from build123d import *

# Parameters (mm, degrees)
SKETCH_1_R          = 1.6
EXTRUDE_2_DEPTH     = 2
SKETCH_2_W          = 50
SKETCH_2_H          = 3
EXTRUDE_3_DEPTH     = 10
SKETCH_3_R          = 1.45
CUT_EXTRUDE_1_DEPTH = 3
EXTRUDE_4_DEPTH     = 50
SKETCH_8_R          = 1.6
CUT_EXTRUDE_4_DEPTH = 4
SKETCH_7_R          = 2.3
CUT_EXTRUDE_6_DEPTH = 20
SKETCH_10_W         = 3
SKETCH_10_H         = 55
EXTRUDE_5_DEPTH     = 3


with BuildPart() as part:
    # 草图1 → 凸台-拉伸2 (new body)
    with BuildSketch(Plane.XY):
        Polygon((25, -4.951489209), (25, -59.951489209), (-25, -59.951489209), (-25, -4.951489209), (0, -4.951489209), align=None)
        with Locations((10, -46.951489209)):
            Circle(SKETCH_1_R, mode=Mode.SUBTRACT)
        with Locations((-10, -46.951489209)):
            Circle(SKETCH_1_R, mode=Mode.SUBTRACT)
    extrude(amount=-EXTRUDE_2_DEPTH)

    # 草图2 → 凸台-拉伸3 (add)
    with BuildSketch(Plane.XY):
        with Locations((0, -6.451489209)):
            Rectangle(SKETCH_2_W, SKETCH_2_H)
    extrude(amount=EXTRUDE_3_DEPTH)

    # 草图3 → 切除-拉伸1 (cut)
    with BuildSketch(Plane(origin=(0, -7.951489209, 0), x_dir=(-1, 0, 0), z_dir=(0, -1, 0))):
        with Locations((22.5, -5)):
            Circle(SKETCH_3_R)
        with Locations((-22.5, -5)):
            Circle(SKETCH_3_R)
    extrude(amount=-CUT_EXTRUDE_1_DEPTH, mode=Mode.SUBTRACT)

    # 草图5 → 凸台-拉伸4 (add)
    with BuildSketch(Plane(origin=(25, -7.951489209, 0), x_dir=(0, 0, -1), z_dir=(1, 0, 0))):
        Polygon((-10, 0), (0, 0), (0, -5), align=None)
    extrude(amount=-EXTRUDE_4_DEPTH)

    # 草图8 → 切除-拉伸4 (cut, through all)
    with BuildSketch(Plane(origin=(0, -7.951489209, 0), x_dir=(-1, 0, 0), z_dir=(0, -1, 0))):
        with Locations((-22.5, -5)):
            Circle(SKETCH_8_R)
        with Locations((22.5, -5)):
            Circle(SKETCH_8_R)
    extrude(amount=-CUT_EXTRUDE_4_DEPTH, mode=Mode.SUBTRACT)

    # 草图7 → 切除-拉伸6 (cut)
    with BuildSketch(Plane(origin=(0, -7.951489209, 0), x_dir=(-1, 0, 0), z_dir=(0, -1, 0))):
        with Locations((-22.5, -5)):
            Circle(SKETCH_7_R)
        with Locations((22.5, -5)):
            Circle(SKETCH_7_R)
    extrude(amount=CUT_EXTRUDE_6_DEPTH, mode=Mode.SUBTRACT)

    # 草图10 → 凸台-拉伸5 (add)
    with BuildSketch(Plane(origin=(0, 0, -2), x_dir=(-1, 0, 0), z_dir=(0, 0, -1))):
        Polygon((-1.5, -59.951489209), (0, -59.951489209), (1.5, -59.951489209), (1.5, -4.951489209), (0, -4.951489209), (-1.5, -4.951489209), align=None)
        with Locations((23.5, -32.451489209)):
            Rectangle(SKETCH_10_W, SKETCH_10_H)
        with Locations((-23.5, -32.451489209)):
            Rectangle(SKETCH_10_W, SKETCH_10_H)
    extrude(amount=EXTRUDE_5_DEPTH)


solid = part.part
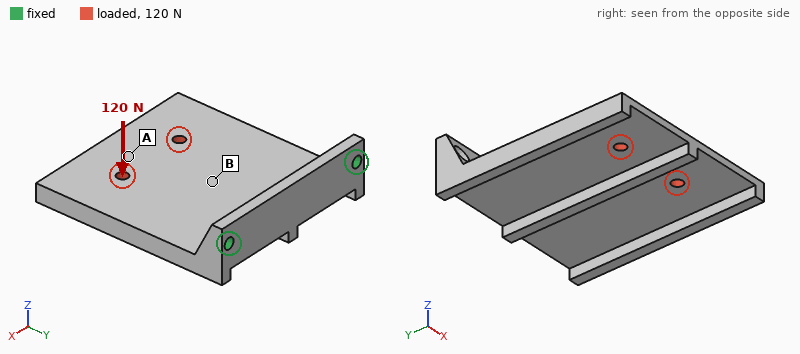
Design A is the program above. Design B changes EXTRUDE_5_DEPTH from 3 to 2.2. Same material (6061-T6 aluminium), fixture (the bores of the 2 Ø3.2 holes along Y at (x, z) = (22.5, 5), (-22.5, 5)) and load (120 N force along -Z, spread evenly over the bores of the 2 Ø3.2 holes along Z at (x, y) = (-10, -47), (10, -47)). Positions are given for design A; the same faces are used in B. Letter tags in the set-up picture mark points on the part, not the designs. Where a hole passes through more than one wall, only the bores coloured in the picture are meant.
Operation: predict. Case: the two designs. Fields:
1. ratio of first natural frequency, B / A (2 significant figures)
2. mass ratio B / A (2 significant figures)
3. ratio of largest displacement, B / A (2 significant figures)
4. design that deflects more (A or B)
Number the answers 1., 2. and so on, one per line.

1. 0.91
2. 0.96
3. 1.3
4. B
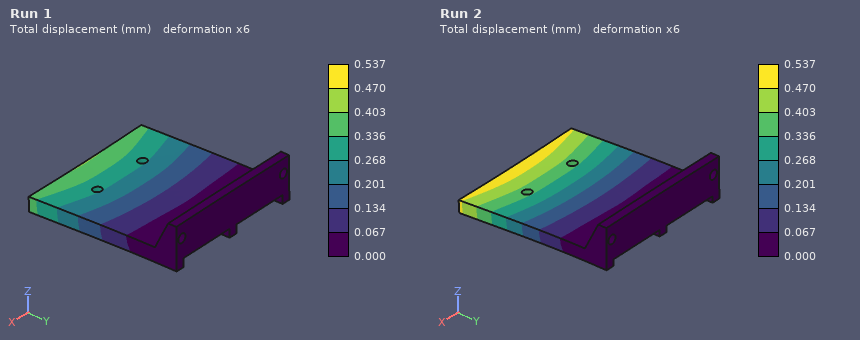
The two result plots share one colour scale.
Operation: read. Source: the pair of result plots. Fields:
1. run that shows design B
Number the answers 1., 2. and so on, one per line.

1. Run 2
